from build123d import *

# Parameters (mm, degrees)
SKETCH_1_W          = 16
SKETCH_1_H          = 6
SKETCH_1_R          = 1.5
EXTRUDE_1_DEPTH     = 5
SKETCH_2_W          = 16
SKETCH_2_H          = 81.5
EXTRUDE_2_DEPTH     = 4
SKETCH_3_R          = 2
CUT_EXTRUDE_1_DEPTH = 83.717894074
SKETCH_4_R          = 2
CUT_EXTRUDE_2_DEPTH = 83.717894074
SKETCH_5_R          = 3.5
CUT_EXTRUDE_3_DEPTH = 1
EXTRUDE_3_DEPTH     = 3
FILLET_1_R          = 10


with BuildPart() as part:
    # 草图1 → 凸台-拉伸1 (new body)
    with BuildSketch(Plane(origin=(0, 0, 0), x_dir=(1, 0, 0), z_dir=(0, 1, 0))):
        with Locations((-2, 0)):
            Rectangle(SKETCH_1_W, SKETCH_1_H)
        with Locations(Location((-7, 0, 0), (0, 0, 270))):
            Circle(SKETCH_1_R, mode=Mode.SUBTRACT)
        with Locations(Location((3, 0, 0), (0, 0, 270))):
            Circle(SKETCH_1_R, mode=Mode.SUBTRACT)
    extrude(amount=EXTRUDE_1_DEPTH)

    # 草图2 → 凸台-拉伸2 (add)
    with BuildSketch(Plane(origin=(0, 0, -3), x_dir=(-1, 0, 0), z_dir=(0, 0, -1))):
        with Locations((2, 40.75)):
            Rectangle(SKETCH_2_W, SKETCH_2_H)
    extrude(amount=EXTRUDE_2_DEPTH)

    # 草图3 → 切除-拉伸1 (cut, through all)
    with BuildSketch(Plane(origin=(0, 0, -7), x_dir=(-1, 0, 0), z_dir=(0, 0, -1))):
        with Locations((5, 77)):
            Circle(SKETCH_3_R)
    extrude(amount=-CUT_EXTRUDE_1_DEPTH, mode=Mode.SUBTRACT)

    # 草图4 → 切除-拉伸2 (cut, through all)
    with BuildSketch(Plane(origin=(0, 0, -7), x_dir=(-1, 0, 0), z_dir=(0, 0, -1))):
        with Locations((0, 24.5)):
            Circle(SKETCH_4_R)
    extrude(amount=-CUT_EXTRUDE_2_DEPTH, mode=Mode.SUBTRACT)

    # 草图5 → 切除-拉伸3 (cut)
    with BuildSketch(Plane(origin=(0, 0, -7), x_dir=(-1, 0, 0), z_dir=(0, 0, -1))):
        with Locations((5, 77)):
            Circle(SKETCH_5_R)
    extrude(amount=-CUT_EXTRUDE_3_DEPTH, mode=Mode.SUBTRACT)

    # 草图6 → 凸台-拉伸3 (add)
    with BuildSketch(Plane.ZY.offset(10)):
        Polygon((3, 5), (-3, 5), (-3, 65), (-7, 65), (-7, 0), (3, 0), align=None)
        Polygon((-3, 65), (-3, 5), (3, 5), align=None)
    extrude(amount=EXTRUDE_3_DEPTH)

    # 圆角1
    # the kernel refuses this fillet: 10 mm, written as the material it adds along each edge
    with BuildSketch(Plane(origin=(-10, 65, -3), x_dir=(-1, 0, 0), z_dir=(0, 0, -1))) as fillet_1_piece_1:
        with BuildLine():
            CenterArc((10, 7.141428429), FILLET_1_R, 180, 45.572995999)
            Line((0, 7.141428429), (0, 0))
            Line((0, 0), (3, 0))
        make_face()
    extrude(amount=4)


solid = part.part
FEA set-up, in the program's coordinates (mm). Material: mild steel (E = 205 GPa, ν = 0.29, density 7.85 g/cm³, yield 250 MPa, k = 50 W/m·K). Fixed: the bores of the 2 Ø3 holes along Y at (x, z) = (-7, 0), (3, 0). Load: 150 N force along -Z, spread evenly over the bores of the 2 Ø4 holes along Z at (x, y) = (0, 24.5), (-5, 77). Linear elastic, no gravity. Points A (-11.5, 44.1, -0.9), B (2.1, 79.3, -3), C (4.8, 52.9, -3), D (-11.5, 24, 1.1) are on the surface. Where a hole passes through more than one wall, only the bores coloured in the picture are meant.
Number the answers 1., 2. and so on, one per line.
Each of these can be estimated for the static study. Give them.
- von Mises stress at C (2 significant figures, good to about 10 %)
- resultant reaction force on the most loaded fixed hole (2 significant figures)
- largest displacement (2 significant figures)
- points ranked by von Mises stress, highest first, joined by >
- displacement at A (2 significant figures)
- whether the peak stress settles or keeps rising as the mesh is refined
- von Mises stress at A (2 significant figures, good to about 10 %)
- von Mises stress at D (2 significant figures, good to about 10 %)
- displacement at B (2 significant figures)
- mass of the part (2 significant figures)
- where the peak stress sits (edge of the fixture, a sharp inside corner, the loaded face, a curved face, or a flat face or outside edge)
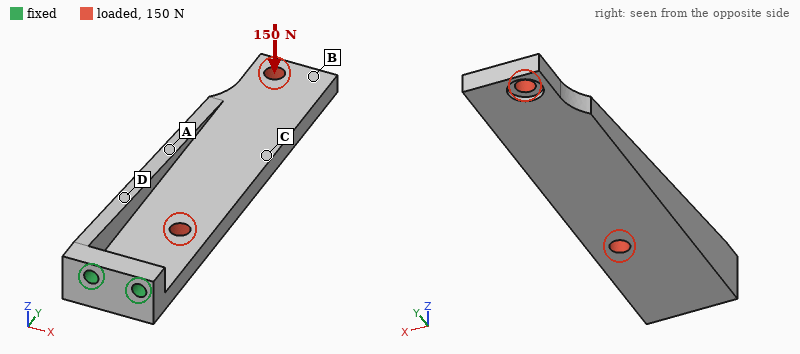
1. 25 MPa
2. 97 N
3. 0.28 mm
4. D > A > C > B
5. 0.089 mm
6. keeps rising
7. 52 MPa
8. 72 MPa
9. 0.26 mm
10. 54 g
11. edge of the fixture
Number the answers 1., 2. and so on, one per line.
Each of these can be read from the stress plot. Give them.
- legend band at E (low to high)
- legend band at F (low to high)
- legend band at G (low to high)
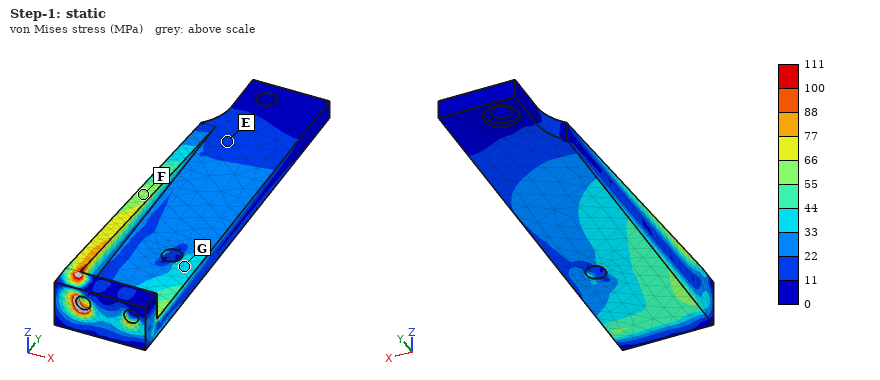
1. 11 to 22 MPa
2. 55 to 66 MPa
3. 33 to 44 MPa
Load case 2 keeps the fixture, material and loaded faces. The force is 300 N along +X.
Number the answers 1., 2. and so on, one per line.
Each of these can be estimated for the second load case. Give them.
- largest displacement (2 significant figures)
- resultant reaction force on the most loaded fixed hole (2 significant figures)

1. 99 µm
2. 970 N
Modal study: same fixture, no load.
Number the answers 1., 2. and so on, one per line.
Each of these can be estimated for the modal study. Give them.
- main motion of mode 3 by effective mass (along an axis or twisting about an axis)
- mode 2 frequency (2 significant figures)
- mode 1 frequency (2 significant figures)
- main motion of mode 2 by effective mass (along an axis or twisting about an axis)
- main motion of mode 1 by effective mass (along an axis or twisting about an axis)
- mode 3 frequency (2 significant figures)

1. along Z
2. 2200 Hz
3. 800 Hz
4. along X
5. along Z
6. 3900 Hz
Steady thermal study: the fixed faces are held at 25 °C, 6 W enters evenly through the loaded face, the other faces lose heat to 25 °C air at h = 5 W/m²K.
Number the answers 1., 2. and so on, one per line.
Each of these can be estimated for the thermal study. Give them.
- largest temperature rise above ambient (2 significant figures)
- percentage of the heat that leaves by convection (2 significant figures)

1. 64 K
2. 12 %
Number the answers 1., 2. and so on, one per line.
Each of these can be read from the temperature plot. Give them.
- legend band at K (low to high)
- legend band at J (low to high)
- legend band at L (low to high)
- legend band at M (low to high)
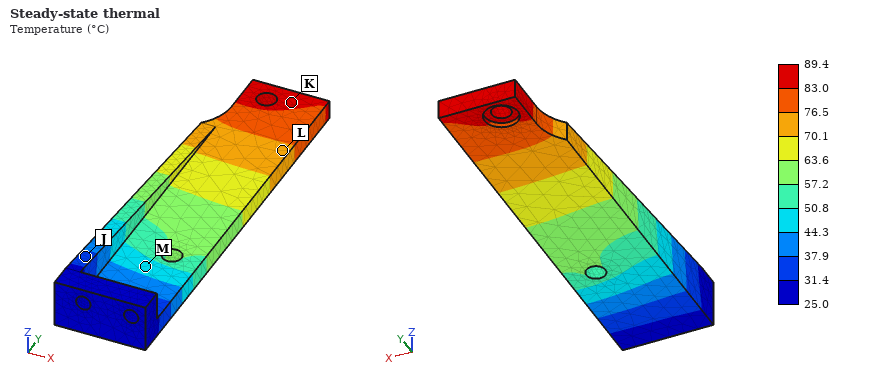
1. 83.0 to 89.4 °C
2. 31.4 to 37.9 °C
3. 70.1 to 76.5 °C
4. 44.3 to 50.8 °C
